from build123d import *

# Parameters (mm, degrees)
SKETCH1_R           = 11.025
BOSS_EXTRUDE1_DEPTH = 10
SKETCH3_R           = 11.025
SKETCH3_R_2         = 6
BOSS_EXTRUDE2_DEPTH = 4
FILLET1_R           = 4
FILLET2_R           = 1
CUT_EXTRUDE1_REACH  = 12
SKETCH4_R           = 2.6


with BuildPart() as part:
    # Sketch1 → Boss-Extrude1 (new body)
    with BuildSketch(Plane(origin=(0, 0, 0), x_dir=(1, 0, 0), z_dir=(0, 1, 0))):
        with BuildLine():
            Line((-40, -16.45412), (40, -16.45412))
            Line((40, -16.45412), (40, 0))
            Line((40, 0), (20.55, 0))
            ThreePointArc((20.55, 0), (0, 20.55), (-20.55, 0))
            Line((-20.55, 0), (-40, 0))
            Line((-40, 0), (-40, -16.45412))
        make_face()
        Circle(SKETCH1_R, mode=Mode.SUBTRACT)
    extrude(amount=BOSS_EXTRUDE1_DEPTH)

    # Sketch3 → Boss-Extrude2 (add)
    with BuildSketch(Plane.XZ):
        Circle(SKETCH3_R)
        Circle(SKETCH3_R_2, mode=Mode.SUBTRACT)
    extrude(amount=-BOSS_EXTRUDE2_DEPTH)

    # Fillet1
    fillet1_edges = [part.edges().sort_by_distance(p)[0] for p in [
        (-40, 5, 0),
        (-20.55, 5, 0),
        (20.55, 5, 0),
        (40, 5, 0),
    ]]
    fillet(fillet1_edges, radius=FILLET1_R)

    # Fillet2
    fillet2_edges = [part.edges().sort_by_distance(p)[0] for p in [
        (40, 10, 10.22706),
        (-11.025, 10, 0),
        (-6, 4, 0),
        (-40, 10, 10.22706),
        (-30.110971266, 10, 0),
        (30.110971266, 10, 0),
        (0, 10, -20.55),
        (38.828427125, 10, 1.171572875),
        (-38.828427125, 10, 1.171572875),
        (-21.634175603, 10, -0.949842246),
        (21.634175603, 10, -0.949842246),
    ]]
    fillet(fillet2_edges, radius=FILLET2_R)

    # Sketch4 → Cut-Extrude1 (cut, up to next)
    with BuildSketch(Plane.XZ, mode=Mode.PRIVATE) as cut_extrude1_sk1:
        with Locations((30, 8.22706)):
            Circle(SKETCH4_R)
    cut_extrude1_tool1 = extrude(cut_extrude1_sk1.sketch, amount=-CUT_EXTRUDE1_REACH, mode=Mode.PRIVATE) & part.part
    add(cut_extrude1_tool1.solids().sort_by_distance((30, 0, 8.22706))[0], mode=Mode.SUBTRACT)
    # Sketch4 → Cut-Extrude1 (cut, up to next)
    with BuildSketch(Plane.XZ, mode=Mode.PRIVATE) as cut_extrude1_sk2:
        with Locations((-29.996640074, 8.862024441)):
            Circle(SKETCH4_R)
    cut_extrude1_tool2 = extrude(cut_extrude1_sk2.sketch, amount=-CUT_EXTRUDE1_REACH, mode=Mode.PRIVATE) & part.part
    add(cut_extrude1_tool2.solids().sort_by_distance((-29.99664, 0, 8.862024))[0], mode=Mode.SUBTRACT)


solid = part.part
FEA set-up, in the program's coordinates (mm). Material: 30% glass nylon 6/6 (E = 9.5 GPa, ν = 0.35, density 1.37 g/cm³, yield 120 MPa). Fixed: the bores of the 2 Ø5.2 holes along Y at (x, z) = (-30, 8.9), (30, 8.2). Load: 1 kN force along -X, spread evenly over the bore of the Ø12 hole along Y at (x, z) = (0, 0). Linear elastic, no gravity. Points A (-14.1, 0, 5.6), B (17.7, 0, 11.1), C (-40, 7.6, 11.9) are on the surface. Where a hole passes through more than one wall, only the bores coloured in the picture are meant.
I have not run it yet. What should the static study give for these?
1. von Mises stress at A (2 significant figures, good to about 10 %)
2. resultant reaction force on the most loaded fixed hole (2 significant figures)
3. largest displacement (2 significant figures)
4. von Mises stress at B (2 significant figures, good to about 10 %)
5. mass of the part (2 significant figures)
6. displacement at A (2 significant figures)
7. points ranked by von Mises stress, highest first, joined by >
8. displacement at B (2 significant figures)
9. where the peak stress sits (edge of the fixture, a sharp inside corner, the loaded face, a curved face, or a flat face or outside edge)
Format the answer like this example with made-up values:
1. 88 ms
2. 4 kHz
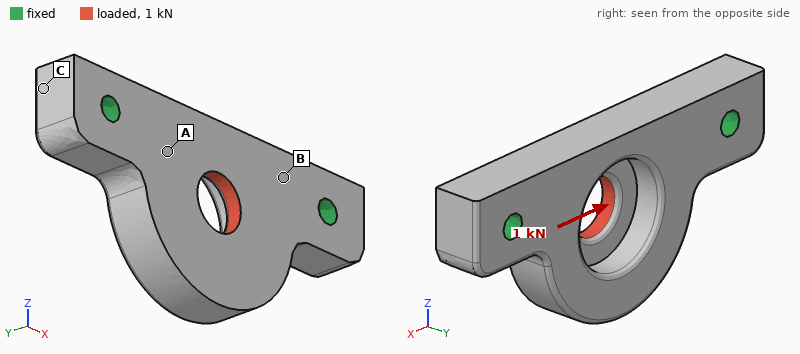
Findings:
1. 6.0 MPa
2. 530 N
3. 22 µm
4. 3.1 MPa
5. 23 g
6. 6.7 µm
7. A > B > C
8. 3.5 µm
9. the loaded face
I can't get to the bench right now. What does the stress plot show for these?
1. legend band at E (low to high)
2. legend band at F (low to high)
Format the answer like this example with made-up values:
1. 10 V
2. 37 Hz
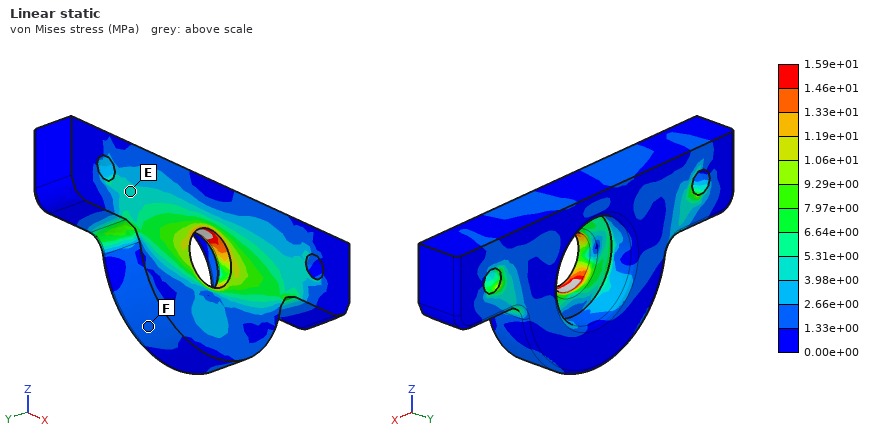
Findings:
1. 3.98e+00 to 5.31e+00 MPa
2. 1.33e+00 to 2.66e+00 MPa
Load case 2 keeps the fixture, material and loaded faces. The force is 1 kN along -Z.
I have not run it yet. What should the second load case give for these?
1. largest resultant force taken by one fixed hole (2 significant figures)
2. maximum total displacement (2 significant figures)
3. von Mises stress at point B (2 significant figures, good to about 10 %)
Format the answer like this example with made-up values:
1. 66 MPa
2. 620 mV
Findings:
1. 520 N
2. 96 µm
3. 7.4 MPa
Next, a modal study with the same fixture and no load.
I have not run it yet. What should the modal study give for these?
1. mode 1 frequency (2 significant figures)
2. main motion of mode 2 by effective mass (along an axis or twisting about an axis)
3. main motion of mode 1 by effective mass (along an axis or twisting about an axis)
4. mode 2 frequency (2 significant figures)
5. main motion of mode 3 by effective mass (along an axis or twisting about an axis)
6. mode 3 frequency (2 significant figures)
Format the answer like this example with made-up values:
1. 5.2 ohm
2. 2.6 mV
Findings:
1. 3300 Hz
2. along Y
3. along Y
4. 7400 Hz
5. along Z
6. 8100 Hz
